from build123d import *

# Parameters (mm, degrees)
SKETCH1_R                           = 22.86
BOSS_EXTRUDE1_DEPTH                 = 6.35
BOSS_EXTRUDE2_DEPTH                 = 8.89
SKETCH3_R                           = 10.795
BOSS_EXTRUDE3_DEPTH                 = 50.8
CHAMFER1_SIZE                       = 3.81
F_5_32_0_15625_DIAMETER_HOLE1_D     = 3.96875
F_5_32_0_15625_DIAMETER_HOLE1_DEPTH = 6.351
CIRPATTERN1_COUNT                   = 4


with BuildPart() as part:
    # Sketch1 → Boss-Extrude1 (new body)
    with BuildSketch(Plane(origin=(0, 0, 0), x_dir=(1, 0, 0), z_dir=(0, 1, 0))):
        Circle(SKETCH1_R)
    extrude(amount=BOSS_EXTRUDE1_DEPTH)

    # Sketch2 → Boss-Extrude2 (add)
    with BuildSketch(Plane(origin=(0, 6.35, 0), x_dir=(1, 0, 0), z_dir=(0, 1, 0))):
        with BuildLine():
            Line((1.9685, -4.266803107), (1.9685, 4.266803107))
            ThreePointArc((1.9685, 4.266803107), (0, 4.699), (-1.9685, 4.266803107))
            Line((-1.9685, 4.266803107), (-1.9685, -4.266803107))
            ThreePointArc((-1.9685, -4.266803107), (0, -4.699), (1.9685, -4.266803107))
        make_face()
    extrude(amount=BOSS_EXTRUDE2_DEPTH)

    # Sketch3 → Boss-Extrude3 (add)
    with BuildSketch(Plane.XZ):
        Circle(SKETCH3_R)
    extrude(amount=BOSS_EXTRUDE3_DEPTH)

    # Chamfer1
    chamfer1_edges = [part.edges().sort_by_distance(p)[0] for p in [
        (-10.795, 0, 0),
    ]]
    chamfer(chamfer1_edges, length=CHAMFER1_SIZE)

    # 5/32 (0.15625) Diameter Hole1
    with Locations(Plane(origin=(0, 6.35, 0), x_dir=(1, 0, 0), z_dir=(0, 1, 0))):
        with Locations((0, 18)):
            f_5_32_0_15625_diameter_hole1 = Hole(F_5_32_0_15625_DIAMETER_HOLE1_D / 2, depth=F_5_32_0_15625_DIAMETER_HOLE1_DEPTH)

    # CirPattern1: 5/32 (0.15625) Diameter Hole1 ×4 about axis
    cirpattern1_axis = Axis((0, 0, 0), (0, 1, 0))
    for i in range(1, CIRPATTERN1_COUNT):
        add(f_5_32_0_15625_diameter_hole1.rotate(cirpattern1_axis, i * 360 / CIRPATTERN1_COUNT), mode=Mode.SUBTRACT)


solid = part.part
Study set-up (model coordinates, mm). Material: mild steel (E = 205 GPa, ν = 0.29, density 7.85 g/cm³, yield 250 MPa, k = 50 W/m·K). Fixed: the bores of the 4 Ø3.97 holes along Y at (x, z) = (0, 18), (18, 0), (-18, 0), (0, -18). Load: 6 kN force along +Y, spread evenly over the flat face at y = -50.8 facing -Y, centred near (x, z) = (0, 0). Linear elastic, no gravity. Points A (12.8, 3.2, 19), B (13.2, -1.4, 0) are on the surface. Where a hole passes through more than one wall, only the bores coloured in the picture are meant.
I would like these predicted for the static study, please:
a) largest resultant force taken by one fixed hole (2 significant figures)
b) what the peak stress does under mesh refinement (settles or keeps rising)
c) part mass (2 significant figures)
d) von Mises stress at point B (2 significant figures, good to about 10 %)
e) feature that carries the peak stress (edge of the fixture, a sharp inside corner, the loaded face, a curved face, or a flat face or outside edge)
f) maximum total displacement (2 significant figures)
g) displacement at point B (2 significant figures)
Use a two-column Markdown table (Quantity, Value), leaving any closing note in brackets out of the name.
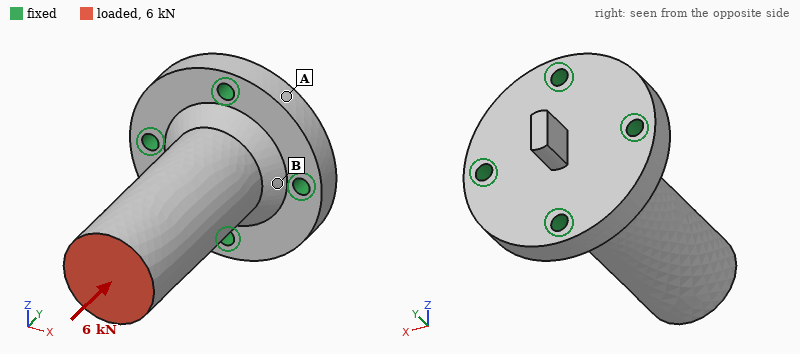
| Quantity | Value |
|---|---|
| largest resultant force taken by one fixed hole | 1.6 kN |
| what the peak stress does under mesh refinement | keeps rising |
| part mass | 230 g |
| von Mises stress at point B | 45 MPa |
| feature that carries the peak stress | edge of the fixture |
| maximum total displacement | 6.5 µm |
| displacement at point B | 1.7 µm |
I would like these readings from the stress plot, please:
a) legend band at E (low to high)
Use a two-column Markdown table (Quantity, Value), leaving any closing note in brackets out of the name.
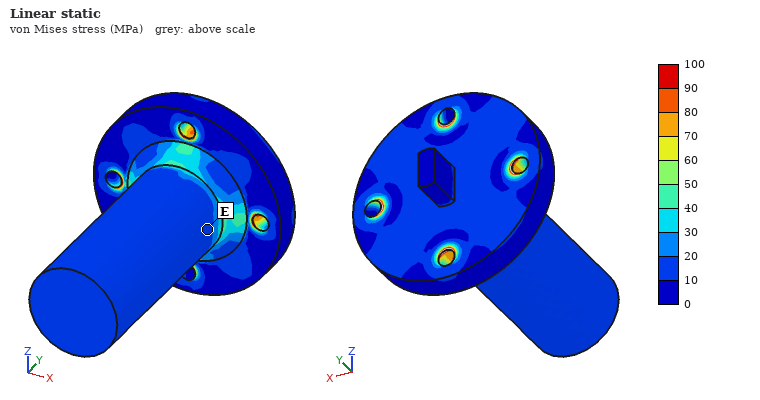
| Quantity | Value |
|---|---|
| legend band at E | 10 to 20 MPa |
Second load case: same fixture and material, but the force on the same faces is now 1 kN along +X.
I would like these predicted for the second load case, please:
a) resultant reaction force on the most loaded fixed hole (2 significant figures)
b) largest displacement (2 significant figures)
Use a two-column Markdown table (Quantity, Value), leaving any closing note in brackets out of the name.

| Quantity | Value |
|---|---|
| resultant reaction force on the most loaded fixed hole | 1.6 kN |
| largest displacement | 30 µm |
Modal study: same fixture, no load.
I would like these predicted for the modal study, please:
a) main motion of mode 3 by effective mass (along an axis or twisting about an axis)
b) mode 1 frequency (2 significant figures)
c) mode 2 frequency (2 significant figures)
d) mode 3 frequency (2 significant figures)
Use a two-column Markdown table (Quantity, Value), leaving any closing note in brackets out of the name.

| Quantity | Value |
|---|---|
| main motion of mode 3 by effective mass | along Y |
| mode 1 frequency | 4500 Hz |
| mode 2 frequency | 4600 Hz |
| mode 3 frequency | 15 kHz |
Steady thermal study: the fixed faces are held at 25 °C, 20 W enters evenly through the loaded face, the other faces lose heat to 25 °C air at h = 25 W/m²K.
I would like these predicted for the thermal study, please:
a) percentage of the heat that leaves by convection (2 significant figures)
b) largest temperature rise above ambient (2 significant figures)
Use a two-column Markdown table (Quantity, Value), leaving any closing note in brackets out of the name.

| Quantity | Value |
|---|---|
| percentage of the heat that leaves by convection | 15 % |
| largest temperature rise above ambient | 58 K |
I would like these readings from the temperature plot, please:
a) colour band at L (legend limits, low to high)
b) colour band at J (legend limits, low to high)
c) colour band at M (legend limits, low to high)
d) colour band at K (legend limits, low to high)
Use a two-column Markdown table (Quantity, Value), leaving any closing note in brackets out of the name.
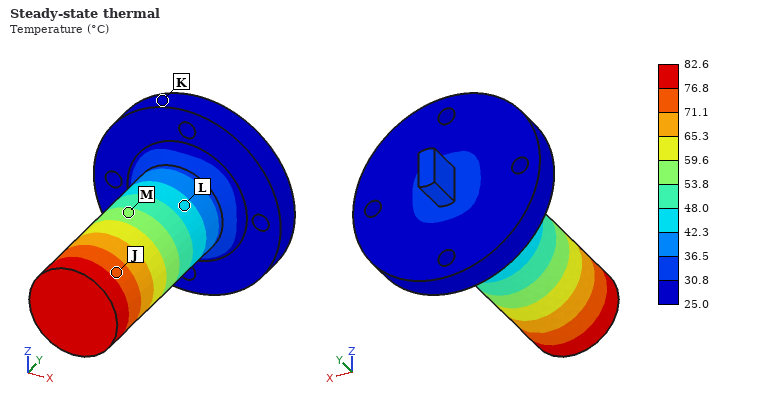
| Quantity | Value |
|---|---|
| colour band at L | 42.3 to 48.0 °C |
| colour band at J | 71.1 to 76.8 °C |
| colour band at M | 53.8 to 59.6 °C |
| colour band at K | 25.0 to 30.8 °C |
